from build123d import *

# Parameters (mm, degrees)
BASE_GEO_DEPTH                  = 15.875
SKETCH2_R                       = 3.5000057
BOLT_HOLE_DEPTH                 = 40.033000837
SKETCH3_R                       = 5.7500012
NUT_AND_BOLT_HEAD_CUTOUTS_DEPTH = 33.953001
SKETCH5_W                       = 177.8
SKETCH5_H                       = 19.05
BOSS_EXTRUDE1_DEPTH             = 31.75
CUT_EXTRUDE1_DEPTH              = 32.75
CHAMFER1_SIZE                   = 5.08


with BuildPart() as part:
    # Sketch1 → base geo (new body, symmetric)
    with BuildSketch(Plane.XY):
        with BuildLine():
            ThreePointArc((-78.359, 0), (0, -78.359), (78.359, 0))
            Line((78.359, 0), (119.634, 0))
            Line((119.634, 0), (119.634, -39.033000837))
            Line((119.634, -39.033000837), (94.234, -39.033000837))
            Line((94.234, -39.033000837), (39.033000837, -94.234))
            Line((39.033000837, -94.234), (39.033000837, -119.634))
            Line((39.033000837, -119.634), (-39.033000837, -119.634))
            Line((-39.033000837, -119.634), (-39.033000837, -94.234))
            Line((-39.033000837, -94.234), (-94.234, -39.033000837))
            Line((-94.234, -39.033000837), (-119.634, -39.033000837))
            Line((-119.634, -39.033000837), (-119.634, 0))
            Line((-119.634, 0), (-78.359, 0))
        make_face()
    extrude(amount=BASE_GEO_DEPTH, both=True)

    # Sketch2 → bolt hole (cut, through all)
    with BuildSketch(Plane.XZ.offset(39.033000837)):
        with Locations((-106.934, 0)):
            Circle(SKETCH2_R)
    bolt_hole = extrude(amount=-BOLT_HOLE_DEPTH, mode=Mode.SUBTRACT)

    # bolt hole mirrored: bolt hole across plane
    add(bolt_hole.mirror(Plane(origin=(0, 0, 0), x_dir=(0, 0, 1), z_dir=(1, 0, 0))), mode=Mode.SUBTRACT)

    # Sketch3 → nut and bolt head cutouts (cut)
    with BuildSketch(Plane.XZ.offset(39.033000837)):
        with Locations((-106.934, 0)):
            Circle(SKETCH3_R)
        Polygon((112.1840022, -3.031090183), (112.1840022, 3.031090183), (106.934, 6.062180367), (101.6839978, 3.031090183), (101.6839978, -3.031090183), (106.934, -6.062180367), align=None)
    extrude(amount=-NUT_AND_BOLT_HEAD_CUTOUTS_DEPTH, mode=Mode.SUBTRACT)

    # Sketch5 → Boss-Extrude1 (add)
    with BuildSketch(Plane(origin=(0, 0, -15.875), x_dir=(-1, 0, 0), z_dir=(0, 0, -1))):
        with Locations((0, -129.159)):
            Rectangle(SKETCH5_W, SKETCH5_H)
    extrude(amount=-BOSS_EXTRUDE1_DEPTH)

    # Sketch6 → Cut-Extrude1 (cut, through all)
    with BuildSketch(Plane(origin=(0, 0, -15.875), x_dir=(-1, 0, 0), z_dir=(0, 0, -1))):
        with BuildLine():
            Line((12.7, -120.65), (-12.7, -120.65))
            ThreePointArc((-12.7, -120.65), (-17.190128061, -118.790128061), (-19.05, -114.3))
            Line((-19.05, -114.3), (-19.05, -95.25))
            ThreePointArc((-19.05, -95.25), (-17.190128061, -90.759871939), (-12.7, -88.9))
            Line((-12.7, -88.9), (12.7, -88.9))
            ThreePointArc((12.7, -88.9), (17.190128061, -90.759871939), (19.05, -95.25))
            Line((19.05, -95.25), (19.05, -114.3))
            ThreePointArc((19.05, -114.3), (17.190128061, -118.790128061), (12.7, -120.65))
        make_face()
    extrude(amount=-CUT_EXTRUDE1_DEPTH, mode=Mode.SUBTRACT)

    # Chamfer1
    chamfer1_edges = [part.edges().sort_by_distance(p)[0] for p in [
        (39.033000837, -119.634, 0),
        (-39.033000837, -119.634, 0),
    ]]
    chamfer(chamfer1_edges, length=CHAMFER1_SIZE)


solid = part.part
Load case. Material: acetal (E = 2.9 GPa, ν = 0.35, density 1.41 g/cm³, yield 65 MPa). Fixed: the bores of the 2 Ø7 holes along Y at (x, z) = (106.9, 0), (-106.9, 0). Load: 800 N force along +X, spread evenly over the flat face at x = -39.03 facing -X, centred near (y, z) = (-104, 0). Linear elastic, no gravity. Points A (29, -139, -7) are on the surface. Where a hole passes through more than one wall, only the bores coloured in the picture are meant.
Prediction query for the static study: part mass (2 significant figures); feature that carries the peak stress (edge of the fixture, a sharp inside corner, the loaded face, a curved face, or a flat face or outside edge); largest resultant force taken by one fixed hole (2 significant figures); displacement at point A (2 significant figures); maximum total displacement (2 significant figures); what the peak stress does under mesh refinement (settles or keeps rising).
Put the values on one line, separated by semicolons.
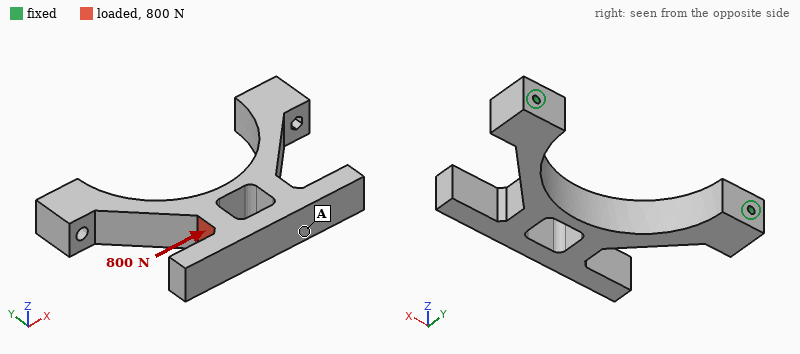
490 g; edge of the fixture; 540 N; 0.16 mm; 0.42 mm; keeps rising
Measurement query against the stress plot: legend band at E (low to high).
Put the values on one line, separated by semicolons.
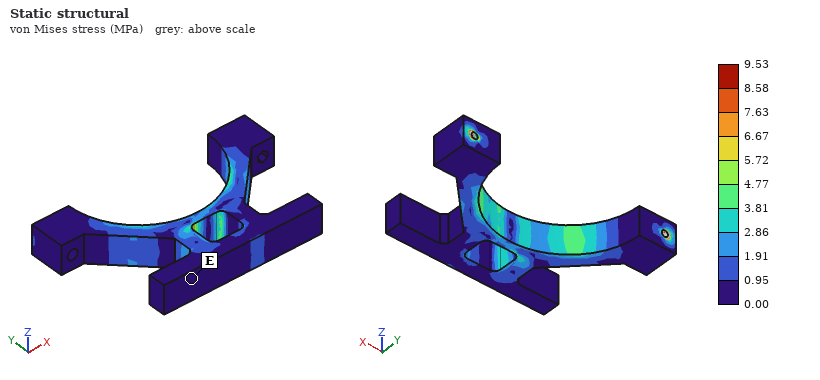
0.00 to 0.95 MPa
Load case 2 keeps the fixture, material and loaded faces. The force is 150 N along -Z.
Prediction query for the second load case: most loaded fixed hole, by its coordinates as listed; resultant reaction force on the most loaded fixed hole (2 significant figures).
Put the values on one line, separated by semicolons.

(-106.9, 0); 100 N
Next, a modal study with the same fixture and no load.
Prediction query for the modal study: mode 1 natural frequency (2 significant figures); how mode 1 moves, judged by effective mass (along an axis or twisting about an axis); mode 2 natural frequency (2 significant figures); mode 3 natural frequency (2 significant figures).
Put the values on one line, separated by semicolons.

78 Hz; along Z; 340 Hz; 350 Hz
